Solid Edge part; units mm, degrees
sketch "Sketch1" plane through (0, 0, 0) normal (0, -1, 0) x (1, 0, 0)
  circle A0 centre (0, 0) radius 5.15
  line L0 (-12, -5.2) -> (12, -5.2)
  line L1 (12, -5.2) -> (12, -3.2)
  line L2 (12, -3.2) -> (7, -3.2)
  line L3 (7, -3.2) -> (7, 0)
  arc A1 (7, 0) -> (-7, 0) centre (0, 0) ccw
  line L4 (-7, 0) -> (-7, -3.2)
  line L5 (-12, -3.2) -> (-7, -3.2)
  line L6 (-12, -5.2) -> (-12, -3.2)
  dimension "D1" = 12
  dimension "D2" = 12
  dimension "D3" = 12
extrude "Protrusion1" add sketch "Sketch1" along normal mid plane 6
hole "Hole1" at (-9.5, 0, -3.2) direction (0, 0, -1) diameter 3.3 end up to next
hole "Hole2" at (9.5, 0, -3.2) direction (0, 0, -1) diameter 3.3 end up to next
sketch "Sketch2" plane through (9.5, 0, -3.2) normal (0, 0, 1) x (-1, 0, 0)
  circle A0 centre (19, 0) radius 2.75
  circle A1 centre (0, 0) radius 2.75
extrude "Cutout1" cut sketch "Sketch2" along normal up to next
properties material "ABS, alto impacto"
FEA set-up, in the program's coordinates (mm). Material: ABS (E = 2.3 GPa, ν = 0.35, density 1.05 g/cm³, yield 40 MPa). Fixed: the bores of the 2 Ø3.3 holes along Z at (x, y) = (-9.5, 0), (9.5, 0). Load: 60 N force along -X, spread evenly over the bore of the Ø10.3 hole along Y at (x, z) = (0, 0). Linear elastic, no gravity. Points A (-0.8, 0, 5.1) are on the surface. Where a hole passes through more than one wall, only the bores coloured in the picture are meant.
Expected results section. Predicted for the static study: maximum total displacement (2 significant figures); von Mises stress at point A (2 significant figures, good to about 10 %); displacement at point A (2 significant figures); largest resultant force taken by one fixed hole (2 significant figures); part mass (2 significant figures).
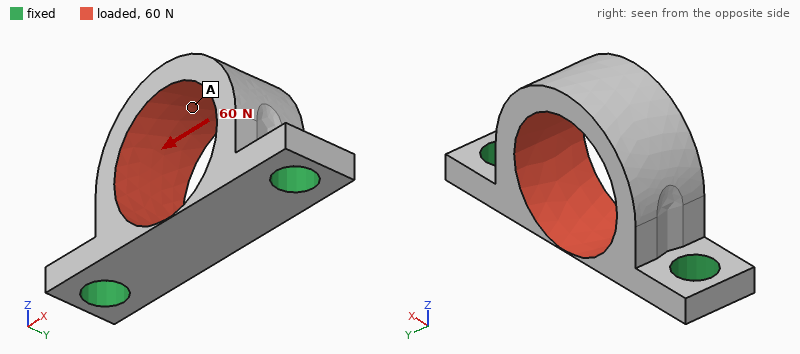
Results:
0.14 mm
3.2 MPa
0.13 mm
32 N
0.51 g
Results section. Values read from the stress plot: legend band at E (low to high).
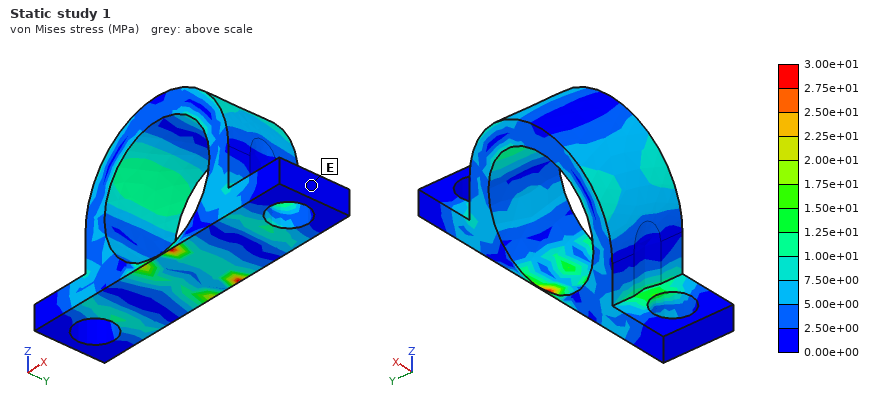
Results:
0.00e+00 to 2.50e+00 MPa
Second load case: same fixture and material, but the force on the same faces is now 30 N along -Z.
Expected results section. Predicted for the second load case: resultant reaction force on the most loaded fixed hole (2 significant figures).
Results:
15 N
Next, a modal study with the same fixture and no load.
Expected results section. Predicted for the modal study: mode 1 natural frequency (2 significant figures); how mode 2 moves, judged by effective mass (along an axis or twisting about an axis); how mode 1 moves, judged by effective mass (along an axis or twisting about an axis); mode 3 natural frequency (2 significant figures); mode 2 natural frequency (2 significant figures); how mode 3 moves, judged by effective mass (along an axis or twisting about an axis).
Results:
4400 Hz
along X
along Y
9100 Hz
5400 Hz
twisting about Z
